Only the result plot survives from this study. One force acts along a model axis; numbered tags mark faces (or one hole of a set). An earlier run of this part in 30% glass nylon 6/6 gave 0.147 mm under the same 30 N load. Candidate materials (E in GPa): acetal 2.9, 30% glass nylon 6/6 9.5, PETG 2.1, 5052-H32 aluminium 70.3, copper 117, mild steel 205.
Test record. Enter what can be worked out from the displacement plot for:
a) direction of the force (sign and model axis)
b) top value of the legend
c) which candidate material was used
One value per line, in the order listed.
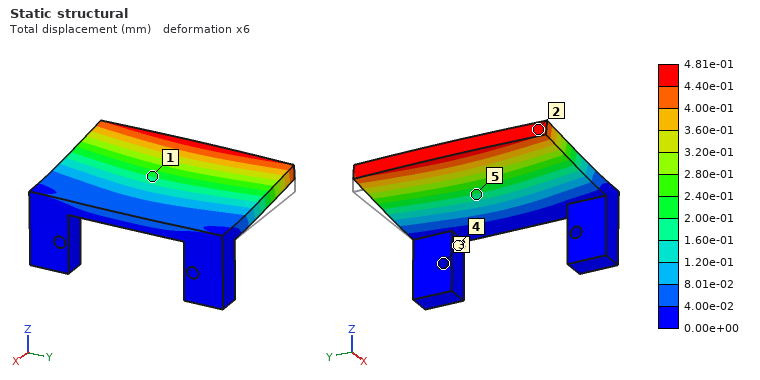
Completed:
+Z
4.81e-01 mm
acetal
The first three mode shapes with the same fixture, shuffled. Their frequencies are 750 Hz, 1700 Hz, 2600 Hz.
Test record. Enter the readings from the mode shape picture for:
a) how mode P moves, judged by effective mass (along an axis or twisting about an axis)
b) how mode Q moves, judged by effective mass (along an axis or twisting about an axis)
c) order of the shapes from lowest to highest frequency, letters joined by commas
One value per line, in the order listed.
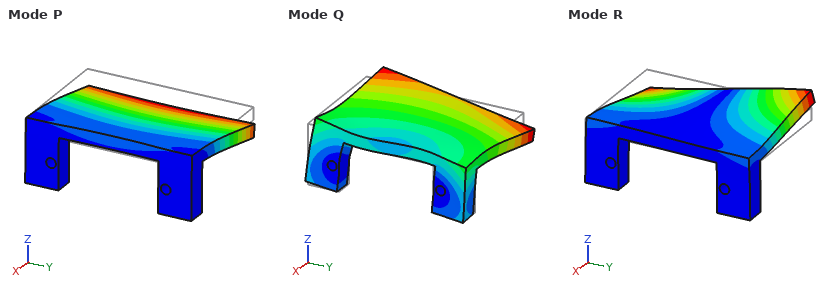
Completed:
along Z
along Y
P, R, Q
